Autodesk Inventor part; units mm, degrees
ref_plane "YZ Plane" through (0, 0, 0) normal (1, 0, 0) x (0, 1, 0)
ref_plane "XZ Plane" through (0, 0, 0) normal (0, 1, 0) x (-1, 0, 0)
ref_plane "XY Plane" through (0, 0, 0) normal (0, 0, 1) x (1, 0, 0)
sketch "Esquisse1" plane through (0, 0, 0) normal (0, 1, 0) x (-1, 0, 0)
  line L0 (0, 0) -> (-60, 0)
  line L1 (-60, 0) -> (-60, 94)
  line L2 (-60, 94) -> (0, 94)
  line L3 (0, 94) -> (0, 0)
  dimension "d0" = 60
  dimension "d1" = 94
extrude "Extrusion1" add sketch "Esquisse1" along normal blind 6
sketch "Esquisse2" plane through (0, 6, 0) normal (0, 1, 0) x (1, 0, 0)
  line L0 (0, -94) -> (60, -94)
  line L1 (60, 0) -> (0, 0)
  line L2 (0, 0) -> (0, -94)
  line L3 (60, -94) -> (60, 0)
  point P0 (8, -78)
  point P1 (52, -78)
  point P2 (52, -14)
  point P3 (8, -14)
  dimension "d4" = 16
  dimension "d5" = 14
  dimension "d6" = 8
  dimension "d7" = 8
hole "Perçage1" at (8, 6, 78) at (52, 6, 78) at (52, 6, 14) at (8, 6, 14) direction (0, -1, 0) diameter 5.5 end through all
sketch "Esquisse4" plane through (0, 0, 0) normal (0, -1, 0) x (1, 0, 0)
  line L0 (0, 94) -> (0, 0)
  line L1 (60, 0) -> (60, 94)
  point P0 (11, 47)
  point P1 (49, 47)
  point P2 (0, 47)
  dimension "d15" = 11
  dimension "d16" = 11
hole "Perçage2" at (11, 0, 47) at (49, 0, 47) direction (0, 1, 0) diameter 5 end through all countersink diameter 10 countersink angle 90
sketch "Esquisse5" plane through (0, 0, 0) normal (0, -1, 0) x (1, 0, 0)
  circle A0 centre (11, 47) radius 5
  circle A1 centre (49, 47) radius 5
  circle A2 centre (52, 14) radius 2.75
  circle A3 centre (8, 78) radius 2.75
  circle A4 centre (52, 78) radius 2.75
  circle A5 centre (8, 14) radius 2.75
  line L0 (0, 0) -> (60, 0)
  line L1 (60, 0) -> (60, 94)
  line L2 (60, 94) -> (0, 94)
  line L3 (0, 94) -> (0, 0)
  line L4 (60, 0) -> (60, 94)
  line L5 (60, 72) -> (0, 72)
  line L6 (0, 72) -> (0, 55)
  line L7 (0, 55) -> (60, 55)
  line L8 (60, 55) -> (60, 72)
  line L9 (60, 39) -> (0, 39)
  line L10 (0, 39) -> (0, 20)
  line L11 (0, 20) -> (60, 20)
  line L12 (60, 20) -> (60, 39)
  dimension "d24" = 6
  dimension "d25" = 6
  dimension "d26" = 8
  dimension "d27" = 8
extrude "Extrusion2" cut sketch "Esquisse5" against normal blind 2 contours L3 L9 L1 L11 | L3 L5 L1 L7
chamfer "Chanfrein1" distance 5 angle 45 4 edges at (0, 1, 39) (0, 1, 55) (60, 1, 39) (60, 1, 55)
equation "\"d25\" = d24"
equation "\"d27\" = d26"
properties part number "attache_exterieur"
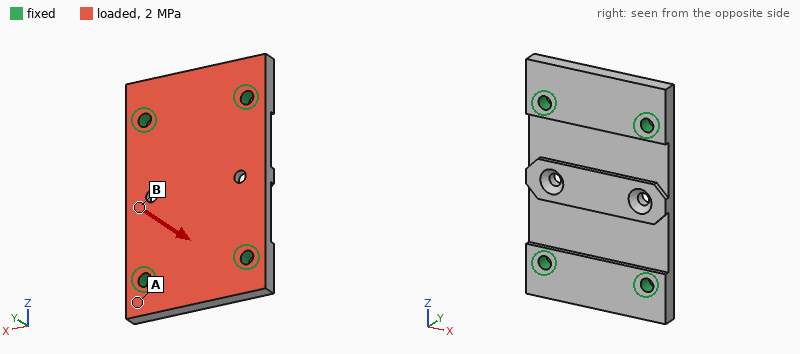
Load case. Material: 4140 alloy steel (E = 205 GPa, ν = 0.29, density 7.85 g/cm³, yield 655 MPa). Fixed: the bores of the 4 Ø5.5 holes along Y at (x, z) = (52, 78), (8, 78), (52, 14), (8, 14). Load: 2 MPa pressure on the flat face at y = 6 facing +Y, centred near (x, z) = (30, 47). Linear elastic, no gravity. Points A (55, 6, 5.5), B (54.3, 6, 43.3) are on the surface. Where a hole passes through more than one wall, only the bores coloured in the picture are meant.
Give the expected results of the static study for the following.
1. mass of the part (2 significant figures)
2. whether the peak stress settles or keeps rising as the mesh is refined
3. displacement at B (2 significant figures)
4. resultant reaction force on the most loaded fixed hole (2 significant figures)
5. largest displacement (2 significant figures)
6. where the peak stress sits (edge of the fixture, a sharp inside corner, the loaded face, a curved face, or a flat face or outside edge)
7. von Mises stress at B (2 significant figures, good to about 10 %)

220 g
keeps rising
47 µm
2.8 kN
51 µm
edge of the fixture
77 MPa
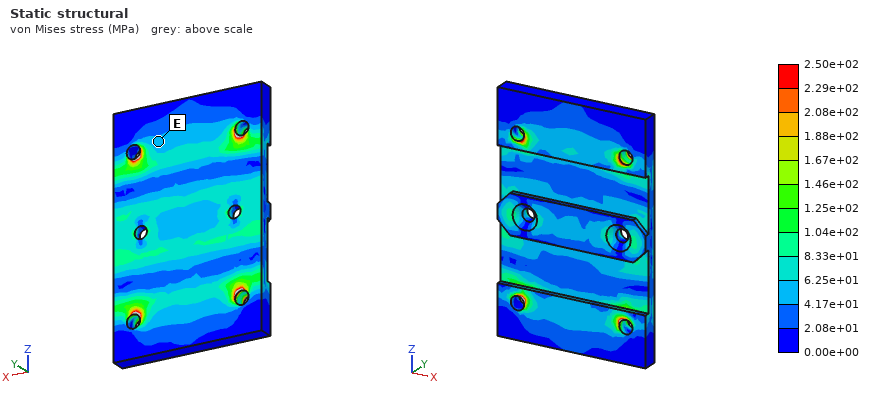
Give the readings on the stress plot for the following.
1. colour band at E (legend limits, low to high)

4.17e+01 to 6.25e+01 MPa
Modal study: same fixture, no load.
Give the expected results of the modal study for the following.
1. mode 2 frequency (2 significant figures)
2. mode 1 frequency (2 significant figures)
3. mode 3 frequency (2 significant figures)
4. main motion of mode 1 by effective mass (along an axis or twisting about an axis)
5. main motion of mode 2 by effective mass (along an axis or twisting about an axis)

7200 Hz
5700 Hz
11 kHz
along Y
twisting about Z
